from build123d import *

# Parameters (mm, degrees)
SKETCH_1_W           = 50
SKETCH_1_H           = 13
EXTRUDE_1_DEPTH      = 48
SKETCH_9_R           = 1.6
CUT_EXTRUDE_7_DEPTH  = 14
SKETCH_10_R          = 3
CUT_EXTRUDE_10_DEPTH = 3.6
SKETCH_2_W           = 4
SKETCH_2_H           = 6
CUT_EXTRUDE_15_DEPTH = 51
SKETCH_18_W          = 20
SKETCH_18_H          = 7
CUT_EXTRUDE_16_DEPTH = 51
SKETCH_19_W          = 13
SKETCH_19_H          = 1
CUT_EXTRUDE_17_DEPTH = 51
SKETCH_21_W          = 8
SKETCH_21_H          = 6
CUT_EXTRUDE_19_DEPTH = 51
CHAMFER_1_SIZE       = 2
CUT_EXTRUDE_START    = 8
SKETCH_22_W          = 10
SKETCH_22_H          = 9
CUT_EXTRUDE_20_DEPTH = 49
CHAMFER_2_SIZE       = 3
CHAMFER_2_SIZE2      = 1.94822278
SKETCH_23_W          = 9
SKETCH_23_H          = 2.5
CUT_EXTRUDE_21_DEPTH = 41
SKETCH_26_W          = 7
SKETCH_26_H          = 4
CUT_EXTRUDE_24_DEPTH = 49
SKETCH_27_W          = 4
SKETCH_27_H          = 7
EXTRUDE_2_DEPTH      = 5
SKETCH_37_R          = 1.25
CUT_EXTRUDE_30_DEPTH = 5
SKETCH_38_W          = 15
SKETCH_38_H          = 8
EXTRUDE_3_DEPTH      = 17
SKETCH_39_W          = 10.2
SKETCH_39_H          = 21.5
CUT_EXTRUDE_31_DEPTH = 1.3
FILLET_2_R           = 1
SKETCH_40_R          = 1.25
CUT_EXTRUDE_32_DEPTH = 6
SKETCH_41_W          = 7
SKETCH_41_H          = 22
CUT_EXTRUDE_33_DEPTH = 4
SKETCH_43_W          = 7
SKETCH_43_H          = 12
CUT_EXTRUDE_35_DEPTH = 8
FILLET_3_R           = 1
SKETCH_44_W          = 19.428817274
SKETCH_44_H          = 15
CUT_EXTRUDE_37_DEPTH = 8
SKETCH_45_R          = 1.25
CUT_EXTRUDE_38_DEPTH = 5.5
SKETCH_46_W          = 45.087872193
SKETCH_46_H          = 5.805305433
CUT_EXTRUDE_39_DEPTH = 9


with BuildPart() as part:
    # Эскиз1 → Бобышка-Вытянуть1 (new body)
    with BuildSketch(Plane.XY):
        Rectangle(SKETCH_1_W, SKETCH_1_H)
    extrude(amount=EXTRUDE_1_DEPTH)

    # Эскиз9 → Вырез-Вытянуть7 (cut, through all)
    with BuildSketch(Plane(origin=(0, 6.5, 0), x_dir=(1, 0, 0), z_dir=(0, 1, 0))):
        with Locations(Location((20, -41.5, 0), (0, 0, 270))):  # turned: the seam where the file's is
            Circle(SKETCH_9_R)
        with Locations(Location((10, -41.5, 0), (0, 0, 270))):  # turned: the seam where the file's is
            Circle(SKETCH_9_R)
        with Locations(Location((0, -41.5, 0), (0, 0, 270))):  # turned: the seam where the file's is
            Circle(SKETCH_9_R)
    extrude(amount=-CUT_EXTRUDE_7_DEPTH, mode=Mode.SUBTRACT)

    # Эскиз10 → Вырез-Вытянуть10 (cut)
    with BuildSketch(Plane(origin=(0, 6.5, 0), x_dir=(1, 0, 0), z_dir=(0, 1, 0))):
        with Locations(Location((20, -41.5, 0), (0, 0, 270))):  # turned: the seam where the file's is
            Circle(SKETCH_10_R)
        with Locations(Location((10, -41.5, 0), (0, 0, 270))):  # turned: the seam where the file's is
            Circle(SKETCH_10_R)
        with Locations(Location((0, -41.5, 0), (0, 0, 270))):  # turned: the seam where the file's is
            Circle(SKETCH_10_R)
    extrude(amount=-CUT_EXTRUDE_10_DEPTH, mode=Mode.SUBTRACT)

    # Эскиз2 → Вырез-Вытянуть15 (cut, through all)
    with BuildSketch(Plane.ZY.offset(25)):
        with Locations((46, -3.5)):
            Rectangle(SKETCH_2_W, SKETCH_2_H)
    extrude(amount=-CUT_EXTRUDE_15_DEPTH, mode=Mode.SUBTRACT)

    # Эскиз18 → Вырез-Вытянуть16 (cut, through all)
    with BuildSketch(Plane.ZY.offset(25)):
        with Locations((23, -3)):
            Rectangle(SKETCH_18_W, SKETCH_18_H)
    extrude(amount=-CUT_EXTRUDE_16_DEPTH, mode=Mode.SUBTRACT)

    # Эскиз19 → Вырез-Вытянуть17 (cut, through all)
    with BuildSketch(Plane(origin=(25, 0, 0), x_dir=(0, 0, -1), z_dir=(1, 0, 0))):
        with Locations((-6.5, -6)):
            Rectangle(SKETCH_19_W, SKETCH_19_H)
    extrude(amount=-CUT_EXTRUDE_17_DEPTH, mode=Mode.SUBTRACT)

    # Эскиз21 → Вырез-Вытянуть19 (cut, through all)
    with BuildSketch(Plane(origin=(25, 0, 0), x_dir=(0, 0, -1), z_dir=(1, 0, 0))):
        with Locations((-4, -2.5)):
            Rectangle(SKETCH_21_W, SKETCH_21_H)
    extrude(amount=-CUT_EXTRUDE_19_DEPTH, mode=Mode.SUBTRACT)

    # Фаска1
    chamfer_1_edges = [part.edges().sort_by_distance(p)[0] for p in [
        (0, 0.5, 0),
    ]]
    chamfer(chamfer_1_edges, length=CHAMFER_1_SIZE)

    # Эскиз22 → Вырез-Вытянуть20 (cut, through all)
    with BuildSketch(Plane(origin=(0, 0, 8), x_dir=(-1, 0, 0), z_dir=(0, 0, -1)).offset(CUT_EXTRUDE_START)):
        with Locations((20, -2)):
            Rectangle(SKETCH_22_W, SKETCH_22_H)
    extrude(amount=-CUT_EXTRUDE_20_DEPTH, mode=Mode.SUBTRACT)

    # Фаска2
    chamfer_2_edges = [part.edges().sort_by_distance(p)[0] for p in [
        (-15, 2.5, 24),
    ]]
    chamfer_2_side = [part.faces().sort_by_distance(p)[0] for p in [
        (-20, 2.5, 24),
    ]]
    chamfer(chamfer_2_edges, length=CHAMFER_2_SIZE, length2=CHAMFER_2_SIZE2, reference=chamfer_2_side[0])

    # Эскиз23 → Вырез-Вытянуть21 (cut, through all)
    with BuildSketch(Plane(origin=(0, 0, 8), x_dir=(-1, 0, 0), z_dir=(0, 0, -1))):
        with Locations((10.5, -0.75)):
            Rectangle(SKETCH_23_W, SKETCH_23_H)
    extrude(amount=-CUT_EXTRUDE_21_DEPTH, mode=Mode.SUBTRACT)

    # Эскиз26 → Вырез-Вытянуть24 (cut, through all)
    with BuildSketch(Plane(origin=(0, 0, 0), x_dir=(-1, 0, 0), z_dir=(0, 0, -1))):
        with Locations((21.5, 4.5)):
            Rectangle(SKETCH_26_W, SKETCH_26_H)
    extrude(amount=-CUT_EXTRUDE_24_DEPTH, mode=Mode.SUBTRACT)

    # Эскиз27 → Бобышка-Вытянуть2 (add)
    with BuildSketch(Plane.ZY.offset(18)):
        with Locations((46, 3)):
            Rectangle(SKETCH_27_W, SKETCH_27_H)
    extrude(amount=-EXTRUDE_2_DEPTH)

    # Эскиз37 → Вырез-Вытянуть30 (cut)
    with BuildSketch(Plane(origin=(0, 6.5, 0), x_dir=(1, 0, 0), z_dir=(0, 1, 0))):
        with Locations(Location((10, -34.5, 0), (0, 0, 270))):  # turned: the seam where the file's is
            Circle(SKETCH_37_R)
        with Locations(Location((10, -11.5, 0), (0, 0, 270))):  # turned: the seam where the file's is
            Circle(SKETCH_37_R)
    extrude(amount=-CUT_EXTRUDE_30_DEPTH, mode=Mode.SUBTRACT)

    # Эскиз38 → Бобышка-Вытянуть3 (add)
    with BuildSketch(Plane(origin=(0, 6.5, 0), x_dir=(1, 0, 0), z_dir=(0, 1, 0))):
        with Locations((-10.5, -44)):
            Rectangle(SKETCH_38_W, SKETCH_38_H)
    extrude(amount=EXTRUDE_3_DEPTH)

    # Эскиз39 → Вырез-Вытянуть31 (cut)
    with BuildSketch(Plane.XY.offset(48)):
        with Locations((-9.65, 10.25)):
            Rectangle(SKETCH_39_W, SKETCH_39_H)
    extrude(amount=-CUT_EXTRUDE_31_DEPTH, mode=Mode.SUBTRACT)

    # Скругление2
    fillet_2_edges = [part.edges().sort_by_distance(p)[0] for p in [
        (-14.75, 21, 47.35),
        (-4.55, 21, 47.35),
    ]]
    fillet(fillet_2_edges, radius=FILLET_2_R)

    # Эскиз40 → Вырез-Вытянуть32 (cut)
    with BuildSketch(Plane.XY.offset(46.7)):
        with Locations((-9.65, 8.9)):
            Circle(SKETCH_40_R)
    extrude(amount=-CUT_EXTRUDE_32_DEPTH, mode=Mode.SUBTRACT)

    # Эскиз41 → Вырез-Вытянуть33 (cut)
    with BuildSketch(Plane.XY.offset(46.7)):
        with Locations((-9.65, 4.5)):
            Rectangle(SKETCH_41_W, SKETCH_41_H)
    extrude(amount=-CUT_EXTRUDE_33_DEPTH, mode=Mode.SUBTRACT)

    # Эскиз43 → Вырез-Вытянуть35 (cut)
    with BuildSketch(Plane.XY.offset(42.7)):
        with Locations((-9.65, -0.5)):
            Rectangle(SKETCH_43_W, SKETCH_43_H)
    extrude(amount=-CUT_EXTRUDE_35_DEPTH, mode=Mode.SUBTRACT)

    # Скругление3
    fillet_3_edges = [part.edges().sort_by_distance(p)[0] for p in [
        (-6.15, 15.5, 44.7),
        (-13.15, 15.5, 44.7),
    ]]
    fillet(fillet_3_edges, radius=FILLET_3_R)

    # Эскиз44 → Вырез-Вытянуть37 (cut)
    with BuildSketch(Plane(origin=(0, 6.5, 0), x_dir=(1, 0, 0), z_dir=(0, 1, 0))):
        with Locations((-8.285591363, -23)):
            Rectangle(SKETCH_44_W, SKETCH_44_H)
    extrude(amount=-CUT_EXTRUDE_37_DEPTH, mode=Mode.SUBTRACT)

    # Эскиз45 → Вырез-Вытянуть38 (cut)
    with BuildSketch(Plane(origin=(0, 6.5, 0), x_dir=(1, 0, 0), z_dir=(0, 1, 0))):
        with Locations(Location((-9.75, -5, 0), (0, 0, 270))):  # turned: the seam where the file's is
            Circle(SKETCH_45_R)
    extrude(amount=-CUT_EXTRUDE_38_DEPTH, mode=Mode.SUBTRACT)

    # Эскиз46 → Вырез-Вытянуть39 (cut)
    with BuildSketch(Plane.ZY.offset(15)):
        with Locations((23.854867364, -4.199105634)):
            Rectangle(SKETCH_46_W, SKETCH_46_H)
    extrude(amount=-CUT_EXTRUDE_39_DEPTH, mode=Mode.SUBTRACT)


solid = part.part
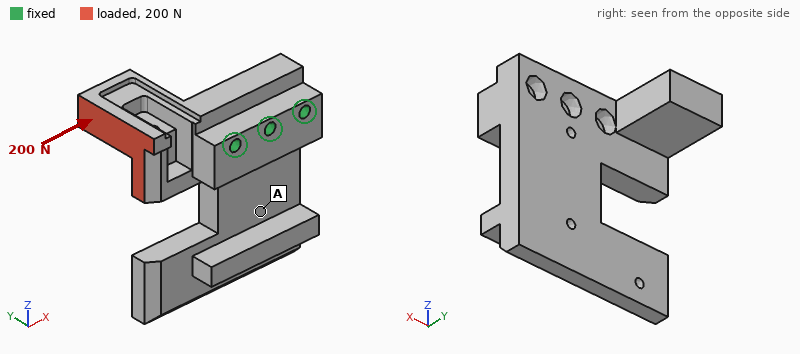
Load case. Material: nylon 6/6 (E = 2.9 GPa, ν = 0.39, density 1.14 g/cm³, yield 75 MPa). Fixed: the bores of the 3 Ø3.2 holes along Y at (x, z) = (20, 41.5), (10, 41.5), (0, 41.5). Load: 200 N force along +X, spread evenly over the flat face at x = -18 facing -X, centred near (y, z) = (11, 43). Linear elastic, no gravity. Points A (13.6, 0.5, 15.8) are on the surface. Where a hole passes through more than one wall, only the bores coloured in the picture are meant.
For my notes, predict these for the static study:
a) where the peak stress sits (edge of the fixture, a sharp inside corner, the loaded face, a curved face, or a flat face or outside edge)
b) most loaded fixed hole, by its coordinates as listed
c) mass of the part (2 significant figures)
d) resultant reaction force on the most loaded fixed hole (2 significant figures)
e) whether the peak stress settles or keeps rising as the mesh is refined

a sharp inside corner
(0, 41.5)
16 g
140 N
keeps rising
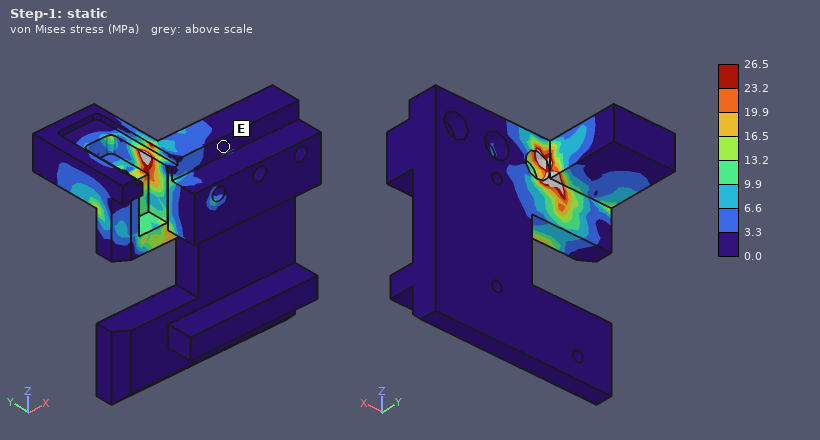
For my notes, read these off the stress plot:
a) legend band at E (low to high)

0.0 to 3.3 MPa
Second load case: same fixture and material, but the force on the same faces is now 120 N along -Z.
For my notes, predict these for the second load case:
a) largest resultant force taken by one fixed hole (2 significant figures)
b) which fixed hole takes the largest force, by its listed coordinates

230 N
(0, 41.5)
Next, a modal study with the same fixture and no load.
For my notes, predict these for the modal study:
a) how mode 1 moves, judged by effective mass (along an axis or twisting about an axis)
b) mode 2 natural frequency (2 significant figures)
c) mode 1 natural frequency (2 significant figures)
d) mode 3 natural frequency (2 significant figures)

along Y
1300 Hz
760 Hz
1500 Hz
